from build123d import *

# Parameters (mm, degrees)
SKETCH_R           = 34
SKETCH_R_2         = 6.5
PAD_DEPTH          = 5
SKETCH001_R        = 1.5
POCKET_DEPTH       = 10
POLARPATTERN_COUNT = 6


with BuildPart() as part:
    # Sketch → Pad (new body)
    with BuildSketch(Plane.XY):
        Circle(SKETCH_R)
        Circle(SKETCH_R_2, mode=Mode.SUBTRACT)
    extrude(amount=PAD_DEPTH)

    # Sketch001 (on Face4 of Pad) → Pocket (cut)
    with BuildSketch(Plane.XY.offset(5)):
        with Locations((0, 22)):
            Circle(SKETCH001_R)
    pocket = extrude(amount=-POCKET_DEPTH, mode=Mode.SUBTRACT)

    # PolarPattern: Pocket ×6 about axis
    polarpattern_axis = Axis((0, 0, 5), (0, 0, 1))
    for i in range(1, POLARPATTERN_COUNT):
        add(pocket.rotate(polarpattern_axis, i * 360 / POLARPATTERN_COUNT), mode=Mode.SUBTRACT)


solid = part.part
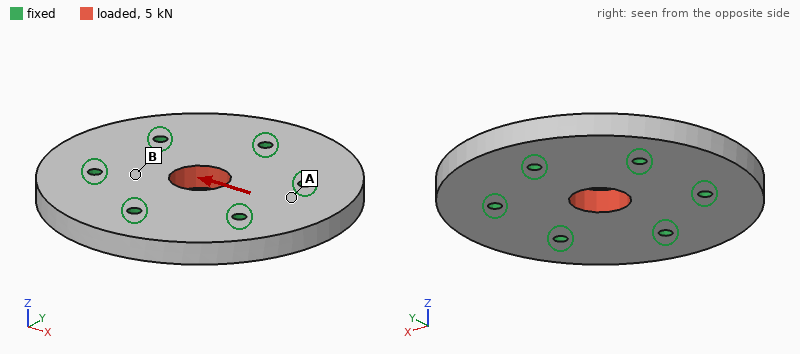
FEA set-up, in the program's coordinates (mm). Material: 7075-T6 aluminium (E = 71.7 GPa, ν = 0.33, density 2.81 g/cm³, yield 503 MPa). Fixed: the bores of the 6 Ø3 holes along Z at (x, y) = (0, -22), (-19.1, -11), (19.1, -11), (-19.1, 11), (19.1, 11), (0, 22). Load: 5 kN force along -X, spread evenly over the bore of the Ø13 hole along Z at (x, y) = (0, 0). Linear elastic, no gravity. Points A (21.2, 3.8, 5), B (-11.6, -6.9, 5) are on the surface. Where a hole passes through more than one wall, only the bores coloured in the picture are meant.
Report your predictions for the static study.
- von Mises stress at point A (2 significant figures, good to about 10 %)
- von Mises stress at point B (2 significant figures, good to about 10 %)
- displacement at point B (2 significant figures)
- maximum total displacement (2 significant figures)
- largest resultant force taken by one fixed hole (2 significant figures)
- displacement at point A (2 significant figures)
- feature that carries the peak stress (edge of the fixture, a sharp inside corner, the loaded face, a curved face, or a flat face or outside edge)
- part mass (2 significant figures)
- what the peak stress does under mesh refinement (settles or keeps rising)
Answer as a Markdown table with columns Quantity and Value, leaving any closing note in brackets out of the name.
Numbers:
| Quantity | Value |
|---|---|
| von Mises stress at point A | 8.1 MPa |
| von Mises stress at point B | 21 MPa |
| displacement at point B | 2.5 µm |
| maximum total displacement | 5.2 µm |
| largest resultant force taken by one fixed hole | 1.1 kN |
| displacement at point A | 1.8 µm |
| feature that carries the peak stress | edge of the fixture |
| part mass | 49 g |
| what the peak stress does under mesh refinement | keeps rising |
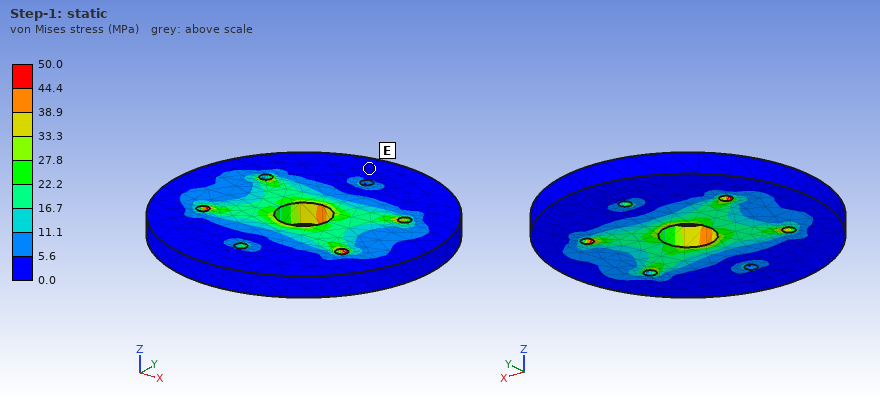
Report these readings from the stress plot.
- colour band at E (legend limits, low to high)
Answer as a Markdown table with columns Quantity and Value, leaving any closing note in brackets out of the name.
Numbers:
| Quantity | Value |
|---|---|
| colour band at E | 0.0 to 5.6 MPa |
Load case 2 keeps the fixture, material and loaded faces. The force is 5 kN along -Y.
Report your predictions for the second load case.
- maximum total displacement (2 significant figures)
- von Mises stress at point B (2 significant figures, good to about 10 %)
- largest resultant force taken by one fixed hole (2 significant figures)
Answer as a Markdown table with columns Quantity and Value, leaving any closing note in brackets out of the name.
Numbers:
| Quantity | Value |
|---|---|
| maximum total displacement | 5.2 µm |
| von Mises stress at point B | 13 MPa |
| largest resultant force taken by one fixed hole | 1.2 kN |
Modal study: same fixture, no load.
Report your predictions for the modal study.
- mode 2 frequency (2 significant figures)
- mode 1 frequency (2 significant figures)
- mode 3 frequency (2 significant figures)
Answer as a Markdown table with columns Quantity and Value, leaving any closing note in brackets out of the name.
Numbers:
| Quantity | Value |
|---|---|
| mode 2 frequency | 18 kHz |
| mode 1 frequency | 17 kHz |
| mode 3 frequency | 18 kHz |
